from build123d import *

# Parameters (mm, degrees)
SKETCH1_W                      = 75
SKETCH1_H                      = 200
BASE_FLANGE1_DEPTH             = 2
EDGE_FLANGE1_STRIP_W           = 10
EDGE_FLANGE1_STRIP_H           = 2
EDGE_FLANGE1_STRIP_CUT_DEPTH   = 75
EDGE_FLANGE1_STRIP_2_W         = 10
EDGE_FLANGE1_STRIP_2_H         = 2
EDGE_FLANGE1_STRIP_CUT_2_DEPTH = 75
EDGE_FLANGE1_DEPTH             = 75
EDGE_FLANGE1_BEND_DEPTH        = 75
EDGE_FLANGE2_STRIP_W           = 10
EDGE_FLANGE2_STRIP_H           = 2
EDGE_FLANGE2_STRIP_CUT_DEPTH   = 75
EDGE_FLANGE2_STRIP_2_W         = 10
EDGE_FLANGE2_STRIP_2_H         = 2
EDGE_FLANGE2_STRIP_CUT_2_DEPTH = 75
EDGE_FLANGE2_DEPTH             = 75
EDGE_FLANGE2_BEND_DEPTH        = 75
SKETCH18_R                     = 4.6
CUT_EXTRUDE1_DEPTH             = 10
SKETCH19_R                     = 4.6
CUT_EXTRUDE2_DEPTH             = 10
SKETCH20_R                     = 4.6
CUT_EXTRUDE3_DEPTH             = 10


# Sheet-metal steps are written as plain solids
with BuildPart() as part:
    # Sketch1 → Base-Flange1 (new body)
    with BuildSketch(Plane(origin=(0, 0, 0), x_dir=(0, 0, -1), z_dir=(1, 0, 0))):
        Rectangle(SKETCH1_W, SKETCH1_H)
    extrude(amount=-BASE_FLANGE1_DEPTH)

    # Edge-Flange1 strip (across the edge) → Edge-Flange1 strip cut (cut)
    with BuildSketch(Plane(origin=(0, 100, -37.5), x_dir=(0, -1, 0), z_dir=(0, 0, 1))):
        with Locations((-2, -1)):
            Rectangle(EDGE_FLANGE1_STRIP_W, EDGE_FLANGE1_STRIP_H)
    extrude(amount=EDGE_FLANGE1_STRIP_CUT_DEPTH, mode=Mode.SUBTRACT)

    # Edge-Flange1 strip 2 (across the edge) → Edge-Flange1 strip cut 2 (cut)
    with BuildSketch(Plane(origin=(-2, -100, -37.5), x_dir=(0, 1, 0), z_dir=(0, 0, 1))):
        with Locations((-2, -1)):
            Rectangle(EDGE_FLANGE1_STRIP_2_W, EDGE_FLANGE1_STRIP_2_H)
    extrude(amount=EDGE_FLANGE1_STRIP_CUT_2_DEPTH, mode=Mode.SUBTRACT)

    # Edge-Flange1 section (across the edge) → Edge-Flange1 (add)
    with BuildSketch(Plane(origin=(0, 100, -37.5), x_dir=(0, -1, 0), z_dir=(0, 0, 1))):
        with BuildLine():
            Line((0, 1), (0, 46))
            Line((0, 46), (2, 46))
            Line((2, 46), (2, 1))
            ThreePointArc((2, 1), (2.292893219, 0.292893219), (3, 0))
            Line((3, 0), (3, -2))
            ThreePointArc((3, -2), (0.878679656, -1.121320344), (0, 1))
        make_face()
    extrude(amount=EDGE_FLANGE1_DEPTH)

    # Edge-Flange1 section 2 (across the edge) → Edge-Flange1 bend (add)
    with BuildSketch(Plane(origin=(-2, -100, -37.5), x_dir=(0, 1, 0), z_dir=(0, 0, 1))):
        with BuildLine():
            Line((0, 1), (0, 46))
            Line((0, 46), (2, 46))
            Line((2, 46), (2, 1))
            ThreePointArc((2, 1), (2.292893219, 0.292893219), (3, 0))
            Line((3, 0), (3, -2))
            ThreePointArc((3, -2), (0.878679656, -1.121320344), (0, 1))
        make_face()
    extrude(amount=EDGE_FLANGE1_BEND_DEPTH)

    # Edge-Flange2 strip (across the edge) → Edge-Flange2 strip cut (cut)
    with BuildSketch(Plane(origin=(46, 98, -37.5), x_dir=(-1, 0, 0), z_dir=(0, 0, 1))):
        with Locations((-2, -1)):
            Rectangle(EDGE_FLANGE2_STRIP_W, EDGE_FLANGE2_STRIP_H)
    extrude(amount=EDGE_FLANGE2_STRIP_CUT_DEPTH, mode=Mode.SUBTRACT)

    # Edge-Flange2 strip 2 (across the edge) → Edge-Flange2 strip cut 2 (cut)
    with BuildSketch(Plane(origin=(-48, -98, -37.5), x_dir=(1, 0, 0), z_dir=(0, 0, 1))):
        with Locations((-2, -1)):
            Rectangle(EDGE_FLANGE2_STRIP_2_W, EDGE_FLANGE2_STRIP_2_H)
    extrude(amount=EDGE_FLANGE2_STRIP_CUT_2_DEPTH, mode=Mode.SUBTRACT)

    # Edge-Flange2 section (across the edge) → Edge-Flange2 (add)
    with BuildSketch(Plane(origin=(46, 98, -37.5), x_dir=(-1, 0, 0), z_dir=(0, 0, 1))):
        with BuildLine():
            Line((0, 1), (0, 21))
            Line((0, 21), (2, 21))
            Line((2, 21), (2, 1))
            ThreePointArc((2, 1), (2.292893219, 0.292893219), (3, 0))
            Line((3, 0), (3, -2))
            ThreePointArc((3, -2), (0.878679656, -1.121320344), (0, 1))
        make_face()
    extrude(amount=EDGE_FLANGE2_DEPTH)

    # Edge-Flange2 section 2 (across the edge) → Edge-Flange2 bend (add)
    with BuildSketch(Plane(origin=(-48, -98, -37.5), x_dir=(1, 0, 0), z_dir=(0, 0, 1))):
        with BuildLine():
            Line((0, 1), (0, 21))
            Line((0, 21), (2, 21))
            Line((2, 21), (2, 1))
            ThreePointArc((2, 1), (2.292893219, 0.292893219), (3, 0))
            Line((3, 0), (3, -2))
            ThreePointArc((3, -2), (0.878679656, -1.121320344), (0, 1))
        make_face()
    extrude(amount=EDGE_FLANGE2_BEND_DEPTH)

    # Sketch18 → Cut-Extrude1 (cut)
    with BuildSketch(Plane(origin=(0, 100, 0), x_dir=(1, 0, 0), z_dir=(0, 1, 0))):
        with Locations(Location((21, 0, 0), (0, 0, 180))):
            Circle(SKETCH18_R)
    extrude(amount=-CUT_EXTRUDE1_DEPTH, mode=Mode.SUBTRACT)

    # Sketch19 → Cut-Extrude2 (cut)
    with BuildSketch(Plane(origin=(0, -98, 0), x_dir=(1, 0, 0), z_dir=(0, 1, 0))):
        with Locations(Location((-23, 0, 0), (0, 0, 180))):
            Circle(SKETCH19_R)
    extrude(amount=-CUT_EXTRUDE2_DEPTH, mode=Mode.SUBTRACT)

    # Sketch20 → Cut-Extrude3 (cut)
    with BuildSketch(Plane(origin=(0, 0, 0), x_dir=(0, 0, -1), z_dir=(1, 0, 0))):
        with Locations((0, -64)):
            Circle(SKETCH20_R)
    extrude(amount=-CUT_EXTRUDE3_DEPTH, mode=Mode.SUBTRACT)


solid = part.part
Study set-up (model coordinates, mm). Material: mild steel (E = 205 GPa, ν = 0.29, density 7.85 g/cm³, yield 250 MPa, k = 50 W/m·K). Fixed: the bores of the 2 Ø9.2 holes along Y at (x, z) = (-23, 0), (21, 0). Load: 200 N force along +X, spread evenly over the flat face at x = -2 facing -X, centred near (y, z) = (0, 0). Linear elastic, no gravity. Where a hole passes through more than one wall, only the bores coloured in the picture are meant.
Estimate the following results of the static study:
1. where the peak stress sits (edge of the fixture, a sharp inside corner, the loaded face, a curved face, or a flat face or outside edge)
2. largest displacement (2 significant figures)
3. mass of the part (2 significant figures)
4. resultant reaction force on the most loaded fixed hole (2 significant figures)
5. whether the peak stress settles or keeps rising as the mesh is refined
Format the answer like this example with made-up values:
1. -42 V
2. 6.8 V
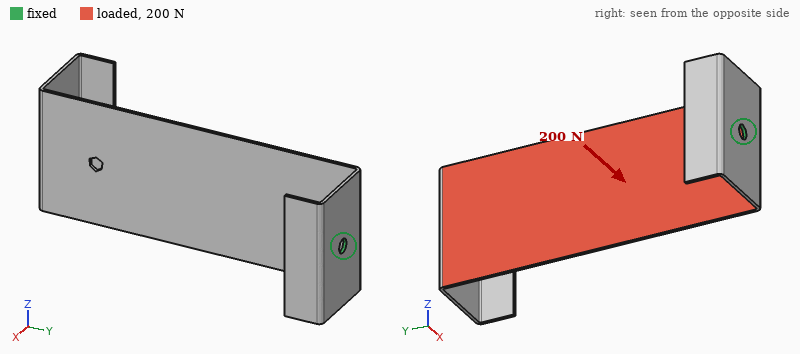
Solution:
1. edge of the fixture
2. 0.69 mm
3. 390 g
4. 100 N
5. keeps rising
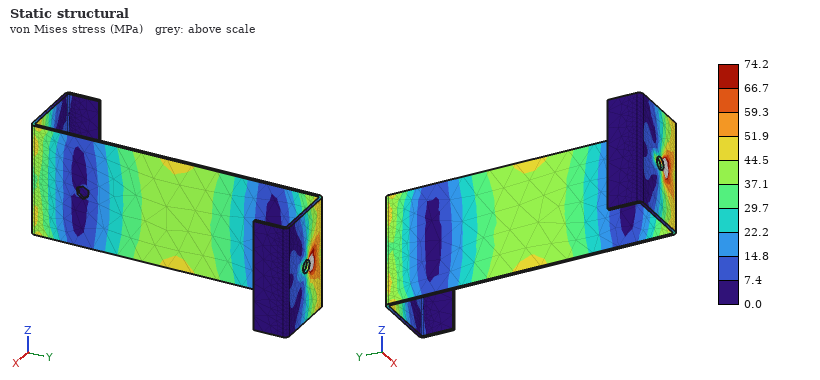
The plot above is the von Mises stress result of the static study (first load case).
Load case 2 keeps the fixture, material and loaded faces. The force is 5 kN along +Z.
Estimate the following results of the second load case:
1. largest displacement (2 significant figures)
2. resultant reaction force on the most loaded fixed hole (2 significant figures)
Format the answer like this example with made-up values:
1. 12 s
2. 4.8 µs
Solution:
1. 0.25 mm
2. 2.5 kN
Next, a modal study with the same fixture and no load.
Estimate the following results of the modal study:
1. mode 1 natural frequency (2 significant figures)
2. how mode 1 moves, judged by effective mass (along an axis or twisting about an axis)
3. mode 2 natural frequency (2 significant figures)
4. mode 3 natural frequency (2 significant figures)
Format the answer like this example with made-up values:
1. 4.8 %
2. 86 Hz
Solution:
1. 210 Hz
2. along X
3. 490 Hz
4. 680 Hz
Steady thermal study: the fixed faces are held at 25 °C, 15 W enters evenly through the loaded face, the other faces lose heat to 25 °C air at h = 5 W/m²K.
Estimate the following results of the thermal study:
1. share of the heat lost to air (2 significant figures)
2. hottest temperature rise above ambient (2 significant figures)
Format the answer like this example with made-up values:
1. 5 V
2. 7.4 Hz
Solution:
1. 32 %
2. 60 K
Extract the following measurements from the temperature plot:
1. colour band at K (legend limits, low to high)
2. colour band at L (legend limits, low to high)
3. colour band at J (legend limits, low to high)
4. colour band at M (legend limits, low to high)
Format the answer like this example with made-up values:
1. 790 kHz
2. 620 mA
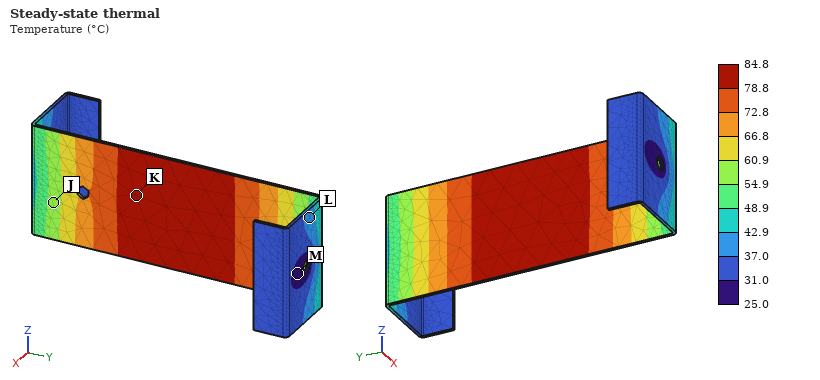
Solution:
1. 78.8 to 84.8 °C
2. 37.0 to 42.9 °C
3. 54.9 to 60.9 °C
4. 25.0 to 31.0 °C
